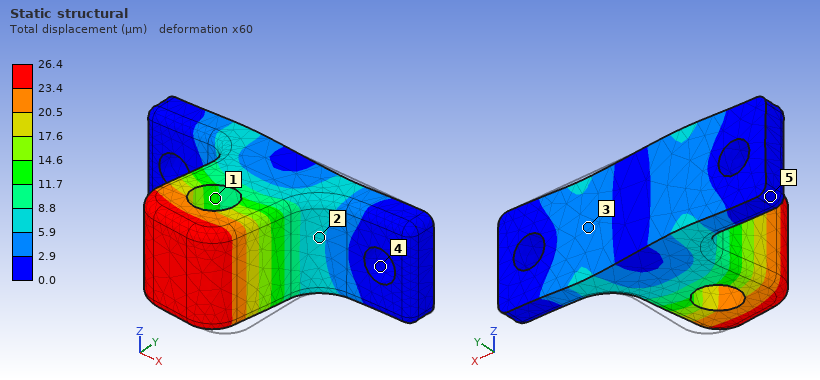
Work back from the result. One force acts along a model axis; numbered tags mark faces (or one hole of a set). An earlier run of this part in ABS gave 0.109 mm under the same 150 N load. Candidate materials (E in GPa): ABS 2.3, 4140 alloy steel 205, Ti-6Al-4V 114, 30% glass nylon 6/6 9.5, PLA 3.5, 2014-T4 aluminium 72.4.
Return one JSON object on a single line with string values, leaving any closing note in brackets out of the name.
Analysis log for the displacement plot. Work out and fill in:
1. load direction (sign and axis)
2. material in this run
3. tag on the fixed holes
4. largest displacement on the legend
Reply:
{"load direction": "-X", "material in this run": "30% glass nylon 6/6", "tag on the fixed holes": "4", "largest displacement on the legend": "26.4 µm"}
